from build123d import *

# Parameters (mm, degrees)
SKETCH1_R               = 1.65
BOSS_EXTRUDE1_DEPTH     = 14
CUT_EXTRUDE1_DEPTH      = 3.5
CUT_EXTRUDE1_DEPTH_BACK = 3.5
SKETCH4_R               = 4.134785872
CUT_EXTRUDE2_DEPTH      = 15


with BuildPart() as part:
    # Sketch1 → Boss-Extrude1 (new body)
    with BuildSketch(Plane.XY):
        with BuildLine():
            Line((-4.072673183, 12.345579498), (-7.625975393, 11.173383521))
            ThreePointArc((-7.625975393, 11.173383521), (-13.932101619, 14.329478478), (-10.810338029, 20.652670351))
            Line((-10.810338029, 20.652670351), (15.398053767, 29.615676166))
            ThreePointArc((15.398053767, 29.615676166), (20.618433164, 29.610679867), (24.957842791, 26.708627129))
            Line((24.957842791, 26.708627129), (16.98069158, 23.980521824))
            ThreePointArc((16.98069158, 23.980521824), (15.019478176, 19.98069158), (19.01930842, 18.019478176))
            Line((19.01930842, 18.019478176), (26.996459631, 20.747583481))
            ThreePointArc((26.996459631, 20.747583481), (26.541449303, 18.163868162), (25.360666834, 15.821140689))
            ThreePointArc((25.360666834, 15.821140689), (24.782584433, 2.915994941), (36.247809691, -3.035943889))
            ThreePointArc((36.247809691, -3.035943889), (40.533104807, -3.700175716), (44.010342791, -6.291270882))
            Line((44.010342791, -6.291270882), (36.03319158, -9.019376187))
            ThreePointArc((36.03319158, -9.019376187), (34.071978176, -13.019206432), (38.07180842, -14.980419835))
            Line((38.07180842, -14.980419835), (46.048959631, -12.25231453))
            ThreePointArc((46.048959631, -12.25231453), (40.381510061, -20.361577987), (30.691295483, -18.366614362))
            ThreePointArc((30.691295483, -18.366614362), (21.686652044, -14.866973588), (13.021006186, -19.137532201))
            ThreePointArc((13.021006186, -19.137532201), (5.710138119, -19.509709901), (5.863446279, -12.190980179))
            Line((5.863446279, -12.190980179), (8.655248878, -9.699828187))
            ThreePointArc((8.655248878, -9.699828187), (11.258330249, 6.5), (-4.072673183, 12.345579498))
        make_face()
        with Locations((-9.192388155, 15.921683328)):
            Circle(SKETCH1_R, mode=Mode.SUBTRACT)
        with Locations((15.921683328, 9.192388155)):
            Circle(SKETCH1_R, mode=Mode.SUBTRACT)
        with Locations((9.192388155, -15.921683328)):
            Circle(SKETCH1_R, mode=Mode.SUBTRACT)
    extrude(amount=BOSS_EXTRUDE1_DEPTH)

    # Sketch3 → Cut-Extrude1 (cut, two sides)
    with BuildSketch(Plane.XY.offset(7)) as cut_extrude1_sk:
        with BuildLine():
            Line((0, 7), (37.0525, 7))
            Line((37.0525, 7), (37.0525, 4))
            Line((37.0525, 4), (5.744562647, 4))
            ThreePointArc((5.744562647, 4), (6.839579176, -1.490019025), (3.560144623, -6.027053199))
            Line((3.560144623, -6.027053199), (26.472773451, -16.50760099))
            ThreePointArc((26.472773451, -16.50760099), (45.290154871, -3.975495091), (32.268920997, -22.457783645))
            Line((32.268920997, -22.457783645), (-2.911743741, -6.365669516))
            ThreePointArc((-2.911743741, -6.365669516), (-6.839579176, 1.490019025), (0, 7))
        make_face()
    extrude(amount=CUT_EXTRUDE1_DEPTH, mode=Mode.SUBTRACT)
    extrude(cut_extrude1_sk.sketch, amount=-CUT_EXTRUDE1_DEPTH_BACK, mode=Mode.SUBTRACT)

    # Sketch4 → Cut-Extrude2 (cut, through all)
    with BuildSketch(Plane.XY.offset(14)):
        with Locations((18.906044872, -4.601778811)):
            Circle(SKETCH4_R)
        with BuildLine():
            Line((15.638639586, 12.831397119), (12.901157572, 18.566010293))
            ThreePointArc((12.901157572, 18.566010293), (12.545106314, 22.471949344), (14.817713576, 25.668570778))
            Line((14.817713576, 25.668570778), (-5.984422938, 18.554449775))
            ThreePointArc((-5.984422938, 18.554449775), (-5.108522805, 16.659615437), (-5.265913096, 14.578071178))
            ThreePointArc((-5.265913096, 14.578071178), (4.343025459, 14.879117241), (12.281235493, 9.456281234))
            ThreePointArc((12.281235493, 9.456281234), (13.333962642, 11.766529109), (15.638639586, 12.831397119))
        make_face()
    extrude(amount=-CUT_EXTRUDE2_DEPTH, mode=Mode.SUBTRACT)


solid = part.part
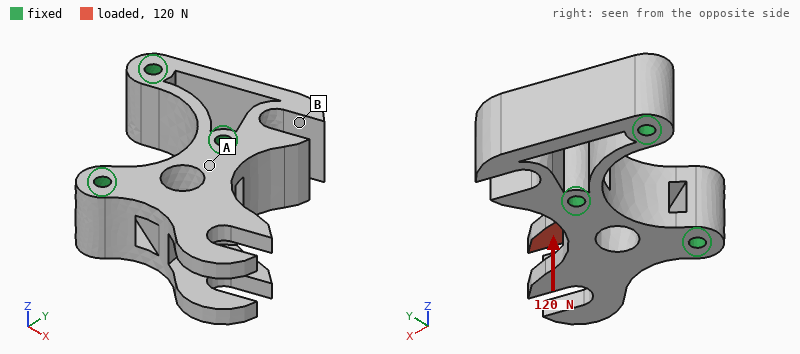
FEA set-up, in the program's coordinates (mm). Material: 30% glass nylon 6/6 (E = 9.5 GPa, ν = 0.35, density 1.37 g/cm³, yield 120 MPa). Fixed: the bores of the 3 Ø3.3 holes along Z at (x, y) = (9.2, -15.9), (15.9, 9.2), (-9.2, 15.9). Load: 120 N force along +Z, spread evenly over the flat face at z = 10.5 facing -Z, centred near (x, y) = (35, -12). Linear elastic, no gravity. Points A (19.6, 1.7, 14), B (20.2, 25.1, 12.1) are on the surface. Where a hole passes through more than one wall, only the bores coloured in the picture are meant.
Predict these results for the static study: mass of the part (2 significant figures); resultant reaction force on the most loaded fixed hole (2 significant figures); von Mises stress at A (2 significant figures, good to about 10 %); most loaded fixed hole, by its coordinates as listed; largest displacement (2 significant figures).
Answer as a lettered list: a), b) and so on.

a) 15 g
b) 67 N
c) 5.3 MPa
d) (9.2, -15.9)
e) 0.40 mm
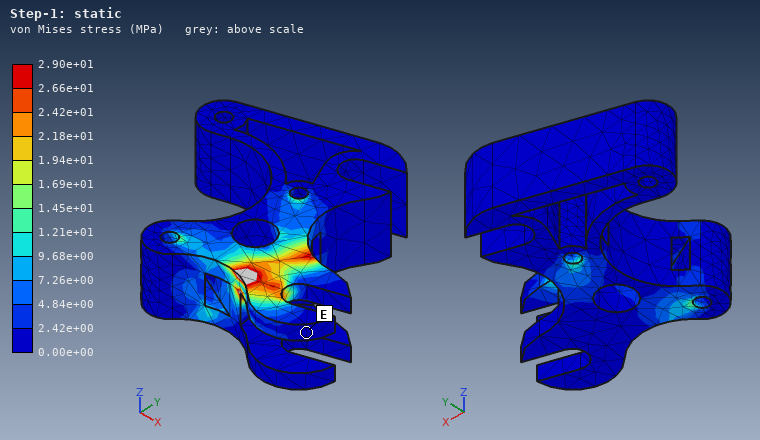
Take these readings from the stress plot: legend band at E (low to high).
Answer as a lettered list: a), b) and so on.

a) 0.00e+00 to 2.42e+00 MPa
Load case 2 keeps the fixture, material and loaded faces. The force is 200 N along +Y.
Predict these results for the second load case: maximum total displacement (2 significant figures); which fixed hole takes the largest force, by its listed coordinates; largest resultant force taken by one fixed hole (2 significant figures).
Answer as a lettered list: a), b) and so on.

a) 0.16 mm
b) (15.9, 9.2)
c) 230 N
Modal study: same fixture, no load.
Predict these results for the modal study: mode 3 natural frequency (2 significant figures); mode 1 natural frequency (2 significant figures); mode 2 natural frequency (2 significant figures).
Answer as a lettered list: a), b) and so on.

a) 6900 Hz
b) 3300 Hz
c) 3700 Hz
